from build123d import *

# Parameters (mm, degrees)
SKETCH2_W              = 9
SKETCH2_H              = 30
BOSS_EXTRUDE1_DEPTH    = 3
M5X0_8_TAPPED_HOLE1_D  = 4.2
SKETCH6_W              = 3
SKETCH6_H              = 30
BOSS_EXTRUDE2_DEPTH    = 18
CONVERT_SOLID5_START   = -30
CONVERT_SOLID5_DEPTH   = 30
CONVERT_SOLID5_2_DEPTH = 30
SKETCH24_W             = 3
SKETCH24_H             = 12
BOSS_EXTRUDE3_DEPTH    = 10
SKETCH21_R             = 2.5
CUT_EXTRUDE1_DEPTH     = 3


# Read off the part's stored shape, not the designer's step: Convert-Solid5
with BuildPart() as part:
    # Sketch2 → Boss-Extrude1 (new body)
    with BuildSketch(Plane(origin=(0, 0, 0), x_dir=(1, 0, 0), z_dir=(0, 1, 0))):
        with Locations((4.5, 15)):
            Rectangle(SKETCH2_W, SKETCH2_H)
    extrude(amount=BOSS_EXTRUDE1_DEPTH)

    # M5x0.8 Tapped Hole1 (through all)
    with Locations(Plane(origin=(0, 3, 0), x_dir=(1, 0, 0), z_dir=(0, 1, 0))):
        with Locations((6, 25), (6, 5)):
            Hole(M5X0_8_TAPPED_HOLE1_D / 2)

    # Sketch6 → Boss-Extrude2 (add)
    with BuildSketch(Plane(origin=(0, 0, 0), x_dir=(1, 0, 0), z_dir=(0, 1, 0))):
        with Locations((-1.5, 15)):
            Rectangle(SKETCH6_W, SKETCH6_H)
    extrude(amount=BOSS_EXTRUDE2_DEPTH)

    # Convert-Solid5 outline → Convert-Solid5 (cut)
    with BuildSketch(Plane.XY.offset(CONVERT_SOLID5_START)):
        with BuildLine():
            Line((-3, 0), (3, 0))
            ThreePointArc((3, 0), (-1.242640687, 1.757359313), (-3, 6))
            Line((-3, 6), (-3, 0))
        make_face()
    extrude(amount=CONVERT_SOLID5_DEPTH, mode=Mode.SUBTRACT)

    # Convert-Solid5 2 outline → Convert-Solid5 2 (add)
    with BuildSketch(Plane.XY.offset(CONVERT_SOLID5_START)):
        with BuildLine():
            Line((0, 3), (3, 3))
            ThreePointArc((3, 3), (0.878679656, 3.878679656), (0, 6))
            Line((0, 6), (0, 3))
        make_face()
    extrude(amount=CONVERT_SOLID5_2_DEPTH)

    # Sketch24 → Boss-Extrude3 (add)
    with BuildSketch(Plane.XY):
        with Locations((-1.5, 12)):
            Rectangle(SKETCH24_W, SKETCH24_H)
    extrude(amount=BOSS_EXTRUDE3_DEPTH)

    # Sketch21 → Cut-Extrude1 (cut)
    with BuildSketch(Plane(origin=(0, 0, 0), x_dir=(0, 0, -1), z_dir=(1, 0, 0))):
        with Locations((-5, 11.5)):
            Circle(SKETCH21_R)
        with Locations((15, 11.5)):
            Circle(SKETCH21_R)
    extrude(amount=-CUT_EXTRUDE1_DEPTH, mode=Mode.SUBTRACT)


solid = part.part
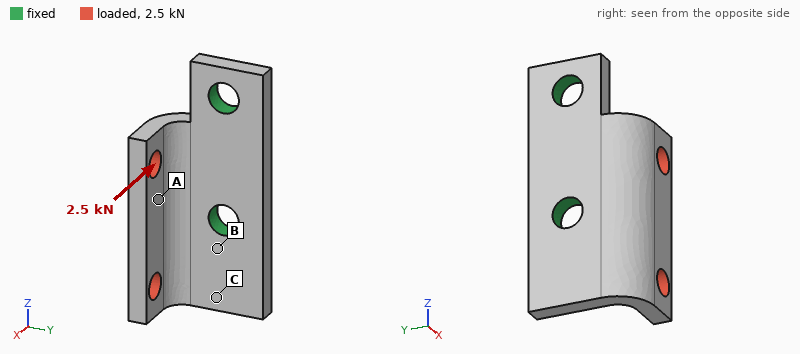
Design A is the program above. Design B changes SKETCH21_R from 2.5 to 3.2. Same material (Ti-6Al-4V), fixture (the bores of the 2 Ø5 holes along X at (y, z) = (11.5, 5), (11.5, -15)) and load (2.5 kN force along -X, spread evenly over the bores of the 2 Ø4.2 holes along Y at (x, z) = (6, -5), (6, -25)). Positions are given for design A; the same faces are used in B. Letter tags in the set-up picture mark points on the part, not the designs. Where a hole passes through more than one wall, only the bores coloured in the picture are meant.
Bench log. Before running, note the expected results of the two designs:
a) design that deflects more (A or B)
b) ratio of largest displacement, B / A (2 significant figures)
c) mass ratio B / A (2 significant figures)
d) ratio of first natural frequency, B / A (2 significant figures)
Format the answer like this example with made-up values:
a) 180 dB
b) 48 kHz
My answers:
a) A
b) 0.81
c) 0.97
d) 1.1
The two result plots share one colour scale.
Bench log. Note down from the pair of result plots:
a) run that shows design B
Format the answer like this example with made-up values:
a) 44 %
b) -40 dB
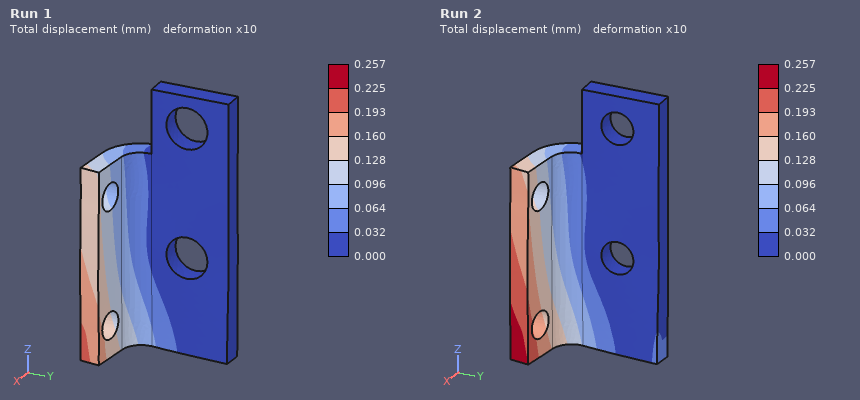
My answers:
a) Run 1
